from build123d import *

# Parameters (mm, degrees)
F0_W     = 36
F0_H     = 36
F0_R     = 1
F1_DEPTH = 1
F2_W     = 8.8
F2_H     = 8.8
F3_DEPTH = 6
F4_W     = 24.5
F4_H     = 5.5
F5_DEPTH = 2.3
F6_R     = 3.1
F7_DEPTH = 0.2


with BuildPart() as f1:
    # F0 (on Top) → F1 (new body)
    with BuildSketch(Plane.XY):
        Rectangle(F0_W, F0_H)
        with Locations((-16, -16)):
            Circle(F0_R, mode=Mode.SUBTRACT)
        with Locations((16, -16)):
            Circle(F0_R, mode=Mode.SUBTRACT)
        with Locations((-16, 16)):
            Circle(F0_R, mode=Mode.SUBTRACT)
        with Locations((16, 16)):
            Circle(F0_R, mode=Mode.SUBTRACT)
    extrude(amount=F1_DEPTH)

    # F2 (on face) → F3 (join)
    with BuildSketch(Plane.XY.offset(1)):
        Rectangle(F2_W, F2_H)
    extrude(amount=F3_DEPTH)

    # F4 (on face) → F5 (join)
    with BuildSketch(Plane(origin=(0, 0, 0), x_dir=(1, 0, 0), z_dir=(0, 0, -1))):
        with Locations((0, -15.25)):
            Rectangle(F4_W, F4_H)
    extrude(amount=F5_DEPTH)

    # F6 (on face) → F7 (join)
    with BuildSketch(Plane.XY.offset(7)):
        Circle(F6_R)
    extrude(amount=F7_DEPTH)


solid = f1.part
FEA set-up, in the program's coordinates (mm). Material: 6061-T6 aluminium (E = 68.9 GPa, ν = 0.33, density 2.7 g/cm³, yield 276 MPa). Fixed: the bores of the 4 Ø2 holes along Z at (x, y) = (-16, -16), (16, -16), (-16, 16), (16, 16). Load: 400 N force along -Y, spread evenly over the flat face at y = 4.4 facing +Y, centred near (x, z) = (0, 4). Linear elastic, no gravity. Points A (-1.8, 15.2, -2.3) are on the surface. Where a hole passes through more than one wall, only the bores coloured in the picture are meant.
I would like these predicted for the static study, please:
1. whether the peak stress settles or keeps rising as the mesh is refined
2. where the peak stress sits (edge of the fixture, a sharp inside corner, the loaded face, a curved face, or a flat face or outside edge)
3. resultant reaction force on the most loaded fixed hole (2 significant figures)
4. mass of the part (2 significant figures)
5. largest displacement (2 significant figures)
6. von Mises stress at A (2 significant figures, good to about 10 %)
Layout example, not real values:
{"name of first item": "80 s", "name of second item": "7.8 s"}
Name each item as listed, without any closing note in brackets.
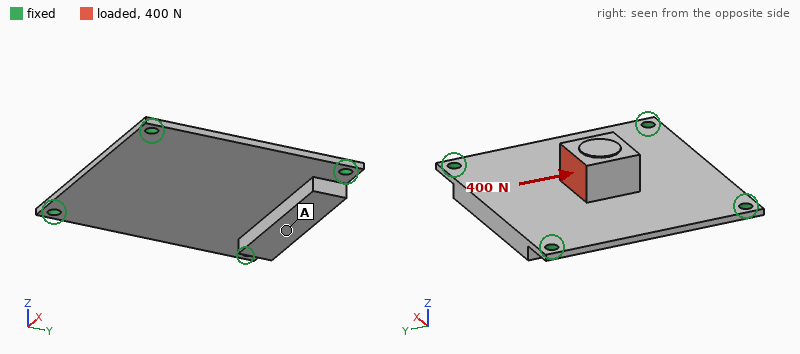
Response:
{"whether the peak stress settles or keeps rising as the mesh is refined": "keeps rising", "where the peak stress sits": "edge of the fixture", "resultant reaction force on the most loaded fixed hole": "110 N", "mass of the part": "5.6 g", "largest displacement": "0.12 mm", "von Mises stress at A": "19 MPa"}
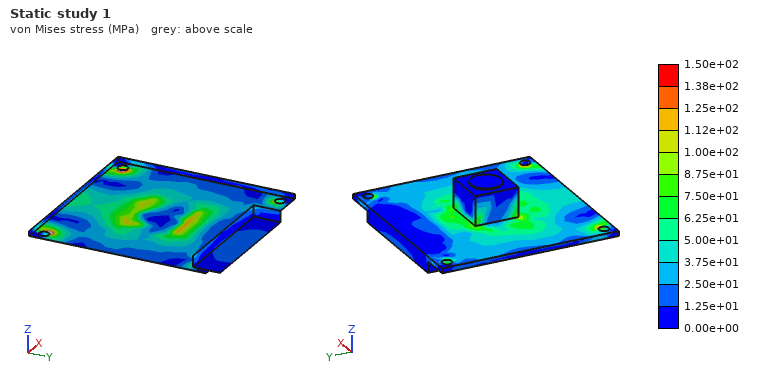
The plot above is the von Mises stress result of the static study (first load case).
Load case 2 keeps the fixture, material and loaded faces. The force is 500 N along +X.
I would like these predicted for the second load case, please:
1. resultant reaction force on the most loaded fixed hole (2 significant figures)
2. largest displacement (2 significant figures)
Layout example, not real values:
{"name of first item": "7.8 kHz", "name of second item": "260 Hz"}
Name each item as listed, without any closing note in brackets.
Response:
{"resultant reaction force on the most loaded fixed hole": "160 N", "largest displacement": "0.13 mm"}
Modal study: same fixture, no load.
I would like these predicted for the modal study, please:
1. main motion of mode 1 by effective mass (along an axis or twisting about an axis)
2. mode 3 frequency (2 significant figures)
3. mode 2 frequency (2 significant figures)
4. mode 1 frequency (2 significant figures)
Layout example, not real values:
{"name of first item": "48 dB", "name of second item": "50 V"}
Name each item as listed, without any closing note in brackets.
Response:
{"main motion of mode 1 by effective mass": "along Z", "mode 3 frequency": "6100 Hz", "mode 2 frequency": "5900 Hz", "mode 1 frequency": "3000 Hz"}
